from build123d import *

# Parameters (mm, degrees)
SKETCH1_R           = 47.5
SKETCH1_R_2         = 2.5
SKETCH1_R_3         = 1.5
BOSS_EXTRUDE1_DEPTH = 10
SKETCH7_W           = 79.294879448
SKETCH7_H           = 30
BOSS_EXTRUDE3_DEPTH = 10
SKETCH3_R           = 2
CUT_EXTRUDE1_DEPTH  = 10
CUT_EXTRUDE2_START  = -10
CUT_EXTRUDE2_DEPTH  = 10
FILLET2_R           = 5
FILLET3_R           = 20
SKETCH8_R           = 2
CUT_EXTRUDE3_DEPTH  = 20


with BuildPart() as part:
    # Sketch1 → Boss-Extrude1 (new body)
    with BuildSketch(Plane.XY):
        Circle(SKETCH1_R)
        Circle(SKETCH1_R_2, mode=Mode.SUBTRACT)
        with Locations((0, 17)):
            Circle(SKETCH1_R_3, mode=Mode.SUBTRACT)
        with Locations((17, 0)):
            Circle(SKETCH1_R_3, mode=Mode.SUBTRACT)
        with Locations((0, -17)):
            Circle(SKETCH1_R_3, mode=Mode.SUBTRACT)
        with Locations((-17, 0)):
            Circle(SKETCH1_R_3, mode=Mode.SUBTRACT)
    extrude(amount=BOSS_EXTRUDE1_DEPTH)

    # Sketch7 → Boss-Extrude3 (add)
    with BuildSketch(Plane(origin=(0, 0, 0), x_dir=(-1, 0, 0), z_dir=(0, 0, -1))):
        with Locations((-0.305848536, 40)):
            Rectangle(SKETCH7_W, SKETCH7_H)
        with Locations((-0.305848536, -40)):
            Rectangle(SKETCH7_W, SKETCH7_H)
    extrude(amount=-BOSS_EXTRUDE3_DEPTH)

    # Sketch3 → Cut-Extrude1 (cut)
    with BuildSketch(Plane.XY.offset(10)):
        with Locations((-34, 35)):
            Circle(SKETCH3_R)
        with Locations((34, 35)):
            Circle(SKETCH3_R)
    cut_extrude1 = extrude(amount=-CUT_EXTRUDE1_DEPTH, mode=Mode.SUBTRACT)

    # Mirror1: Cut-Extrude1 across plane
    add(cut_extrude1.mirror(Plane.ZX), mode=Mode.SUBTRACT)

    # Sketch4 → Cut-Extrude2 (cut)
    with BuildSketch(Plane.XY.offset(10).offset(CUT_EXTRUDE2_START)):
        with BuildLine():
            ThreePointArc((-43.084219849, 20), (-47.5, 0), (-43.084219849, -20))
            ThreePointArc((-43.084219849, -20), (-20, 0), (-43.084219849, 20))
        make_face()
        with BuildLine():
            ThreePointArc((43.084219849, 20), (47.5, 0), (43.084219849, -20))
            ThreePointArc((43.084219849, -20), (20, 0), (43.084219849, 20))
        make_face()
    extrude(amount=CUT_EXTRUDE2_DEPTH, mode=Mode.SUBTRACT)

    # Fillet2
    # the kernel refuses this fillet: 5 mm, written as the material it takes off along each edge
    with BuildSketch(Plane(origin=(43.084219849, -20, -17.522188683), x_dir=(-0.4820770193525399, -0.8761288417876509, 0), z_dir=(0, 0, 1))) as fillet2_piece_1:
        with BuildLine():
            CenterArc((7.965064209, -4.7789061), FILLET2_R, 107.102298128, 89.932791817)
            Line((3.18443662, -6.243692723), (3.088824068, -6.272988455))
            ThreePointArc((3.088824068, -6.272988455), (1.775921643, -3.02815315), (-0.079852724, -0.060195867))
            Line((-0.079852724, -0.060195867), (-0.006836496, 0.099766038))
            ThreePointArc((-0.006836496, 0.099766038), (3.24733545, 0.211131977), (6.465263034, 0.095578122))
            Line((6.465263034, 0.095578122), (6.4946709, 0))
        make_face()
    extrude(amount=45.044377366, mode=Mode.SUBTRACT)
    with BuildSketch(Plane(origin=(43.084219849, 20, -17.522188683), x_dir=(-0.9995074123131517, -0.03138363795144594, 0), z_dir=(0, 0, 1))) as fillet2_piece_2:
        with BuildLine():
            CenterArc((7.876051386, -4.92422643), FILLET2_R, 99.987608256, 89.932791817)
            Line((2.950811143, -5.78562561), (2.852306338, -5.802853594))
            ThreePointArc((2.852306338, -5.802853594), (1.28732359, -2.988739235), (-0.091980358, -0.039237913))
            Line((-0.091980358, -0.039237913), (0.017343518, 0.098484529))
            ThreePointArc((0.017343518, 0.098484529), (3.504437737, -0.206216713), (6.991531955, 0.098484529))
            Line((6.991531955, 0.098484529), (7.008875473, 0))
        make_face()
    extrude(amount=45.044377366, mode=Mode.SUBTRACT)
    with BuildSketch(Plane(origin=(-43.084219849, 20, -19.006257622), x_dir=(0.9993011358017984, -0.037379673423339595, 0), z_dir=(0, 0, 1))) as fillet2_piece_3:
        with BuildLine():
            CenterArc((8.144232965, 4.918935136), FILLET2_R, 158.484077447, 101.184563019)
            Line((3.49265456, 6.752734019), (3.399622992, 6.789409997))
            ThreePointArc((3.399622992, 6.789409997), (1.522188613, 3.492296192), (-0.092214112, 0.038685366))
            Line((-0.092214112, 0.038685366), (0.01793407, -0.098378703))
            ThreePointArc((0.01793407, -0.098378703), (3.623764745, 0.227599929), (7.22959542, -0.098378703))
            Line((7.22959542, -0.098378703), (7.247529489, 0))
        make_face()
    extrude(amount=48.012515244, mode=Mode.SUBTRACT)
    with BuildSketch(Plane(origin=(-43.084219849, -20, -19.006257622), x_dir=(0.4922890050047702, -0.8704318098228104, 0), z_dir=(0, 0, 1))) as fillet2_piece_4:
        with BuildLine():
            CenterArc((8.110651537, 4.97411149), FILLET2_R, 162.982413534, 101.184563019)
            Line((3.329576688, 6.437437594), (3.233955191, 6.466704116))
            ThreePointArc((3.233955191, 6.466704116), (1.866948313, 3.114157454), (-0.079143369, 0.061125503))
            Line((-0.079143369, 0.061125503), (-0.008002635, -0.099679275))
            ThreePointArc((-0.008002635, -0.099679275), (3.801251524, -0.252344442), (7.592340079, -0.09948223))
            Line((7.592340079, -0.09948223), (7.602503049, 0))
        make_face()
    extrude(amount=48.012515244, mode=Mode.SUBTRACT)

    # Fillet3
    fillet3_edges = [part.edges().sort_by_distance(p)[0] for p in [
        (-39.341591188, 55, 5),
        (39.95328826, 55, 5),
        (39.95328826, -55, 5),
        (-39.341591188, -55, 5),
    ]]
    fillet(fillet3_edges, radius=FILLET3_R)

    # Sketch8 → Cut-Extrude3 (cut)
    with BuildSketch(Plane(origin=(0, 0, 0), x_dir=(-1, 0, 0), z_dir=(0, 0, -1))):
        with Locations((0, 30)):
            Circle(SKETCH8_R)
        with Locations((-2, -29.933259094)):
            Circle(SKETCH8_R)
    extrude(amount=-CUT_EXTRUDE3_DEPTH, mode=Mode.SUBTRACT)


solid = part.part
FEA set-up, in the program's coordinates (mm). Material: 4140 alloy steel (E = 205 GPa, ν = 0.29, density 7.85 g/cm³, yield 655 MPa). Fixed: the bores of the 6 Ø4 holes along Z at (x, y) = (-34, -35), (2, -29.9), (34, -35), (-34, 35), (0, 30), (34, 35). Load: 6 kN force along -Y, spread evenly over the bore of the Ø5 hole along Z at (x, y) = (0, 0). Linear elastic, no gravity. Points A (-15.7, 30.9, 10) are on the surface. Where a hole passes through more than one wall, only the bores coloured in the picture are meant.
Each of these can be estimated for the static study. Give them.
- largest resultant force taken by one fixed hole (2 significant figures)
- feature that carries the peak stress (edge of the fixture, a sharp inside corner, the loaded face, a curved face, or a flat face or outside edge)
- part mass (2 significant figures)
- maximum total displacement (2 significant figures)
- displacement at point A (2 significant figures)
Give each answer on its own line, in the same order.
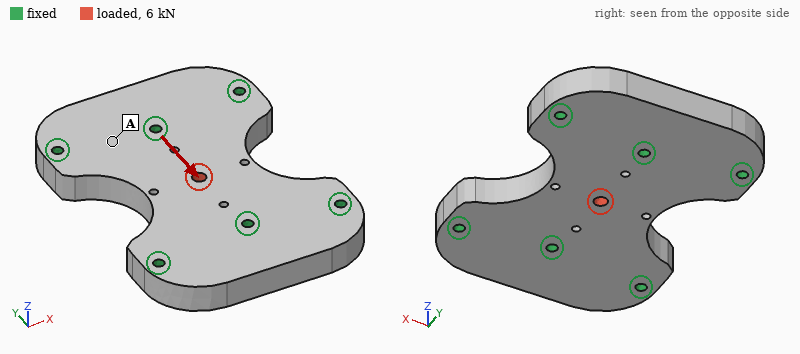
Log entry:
1.8 kN
the loaded face
550 g
2.3 µm
0.39 µm
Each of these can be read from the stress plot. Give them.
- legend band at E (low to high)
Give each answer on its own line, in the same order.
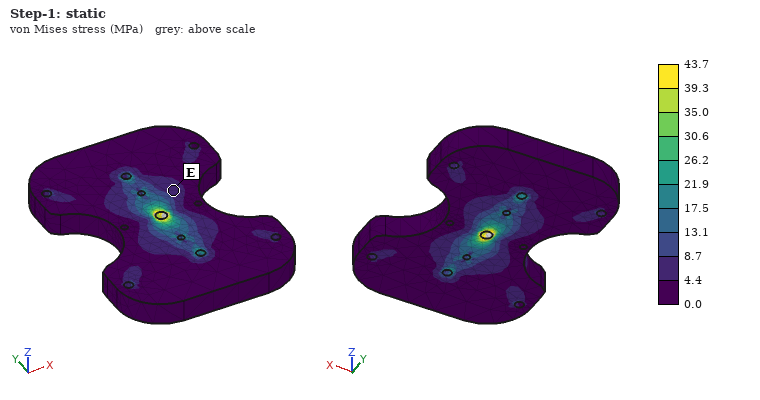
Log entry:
4.4 to 8.7 MPa
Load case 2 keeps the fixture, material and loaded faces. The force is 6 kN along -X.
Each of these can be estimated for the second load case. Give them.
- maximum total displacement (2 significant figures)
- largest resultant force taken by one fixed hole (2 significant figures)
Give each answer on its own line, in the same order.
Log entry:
3.5 µm
1.6 kN
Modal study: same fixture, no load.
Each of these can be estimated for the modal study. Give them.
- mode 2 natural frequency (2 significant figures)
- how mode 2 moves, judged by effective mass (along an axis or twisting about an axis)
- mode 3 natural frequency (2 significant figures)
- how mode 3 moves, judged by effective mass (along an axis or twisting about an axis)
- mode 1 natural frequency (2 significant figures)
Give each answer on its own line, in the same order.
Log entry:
12 kHz
twisting about X
13 kHz
along Z
9800 Hz
